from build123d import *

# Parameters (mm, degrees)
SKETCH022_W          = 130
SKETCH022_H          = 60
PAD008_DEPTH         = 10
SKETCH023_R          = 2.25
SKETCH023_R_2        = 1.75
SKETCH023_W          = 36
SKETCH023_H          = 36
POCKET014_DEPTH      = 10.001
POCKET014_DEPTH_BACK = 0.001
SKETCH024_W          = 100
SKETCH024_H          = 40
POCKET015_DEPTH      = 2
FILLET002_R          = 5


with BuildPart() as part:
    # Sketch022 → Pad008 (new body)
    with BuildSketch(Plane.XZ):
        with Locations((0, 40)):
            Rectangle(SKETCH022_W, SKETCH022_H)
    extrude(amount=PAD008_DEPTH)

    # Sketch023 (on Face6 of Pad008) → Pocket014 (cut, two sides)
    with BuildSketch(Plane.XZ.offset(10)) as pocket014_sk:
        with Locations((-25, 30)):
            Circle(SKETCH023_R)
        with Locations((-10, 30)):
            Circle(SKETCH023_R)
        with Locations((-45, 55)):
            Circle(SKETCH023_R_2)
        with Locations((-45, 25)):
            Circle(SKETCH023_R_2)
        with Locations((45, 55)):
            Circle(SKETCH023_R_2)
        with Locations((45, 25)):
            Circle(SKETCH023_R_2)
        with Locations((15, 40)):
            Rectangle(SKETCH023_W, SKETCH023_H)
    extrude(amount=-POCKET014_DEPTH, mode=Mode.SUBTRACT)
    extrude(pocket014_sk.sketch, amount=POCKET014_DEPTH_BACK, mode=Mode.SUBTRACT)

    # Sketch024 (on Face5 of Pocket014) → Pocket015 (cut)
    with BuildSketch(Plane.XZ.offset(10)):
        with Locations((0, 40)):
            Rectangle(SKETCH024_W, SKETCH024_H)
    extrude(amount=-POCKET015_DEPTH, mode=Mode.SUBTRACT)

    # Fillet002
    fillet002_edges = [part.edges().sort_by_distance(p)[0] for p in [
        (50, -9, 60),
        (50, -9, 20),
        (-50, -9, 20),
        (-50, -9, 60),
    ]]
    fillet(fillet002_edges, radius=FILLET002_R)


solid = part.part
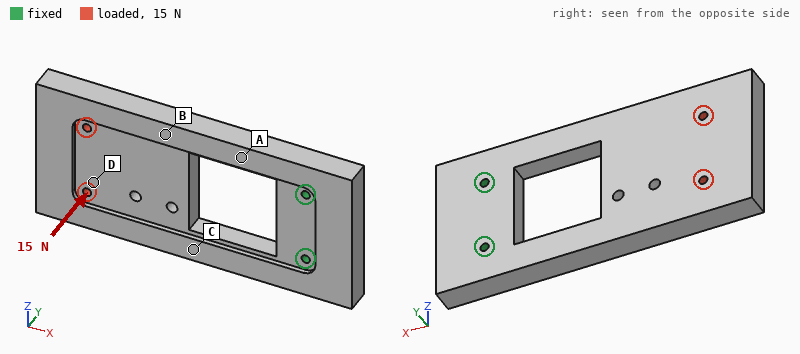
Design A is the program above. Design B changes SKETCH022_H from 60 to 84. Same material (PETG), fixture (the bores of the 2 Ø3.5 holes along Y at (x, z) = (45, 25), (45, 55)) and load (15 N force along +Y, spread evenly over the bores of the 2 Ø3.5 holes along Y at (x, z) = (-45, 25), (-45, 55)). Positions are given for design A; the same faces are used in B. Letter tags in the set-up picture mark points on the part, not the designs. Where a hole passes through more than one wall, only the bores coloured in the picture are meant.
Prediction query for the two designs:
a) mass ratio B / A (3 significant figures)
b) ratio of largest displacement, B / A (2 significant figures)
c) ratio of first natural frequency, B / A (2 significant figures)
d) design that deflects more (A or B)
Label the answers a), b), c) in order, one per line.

a) 1.53
b) 0.62
c) 1.0
d) A
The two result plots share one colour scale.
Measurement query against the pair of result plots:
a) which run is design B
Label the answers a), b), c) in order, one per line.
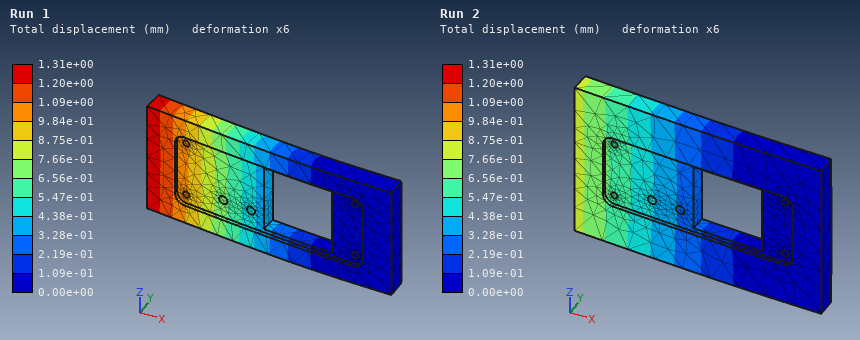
a) Run 2
